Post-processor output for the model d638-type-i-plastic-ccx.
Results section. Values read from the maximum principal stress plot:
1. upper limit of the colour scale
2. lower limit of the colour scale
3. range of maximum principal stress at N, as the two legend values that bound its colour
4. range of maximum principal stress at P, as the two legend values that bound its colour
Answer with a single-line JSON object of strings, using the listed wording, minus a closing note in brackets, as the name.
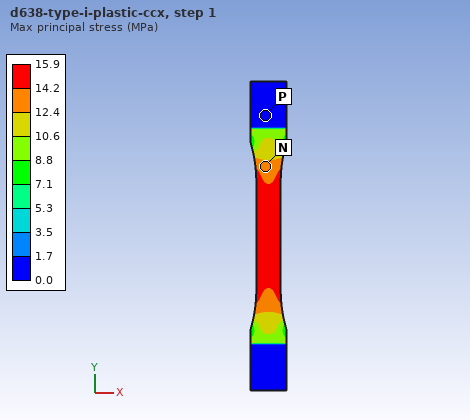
{"upper limit of the colour scale": "15.9 MPa", "lower limit of the colour scale": "0.0 MPa", "range of maximum principal stress at N, as the two legend values that bound its colour": "12.4 to 14.2 MPa", "range of maximum principal stress at P, as the two legend values that bound its colour": "0.0 to 1.7 MPa"}
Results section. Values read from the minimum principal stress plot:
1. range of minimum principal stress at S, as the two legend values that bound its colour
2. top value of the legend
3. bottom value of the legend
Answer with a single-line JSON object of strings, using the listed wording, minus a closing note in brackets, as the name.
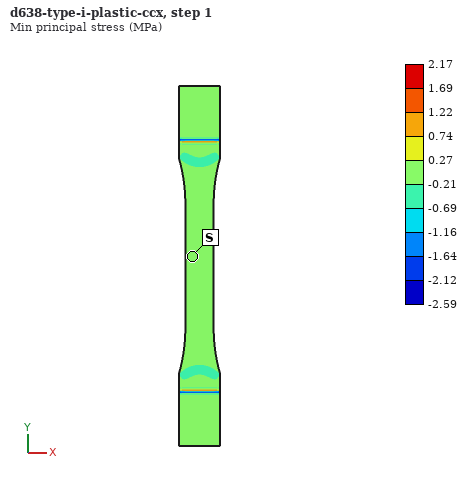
{"range of minimum principal stress at S, as the two legend values that bound its colour": "-0.21 to 0.27 MPa", "top value of the legend": "2.17 MPa", "bottom value of the legend": "-2.59 MPa"}
